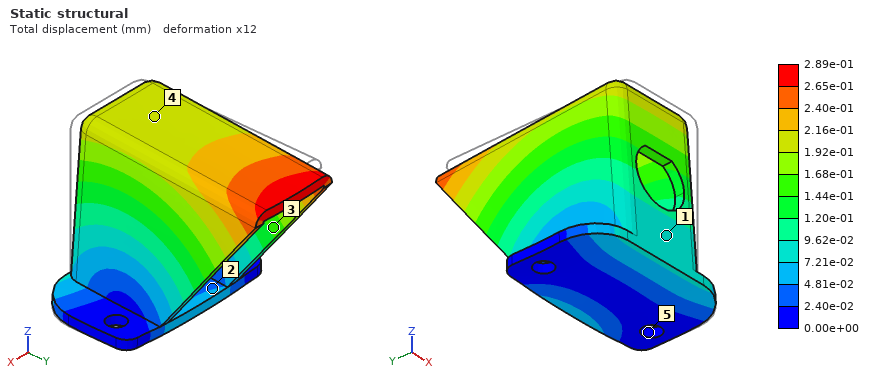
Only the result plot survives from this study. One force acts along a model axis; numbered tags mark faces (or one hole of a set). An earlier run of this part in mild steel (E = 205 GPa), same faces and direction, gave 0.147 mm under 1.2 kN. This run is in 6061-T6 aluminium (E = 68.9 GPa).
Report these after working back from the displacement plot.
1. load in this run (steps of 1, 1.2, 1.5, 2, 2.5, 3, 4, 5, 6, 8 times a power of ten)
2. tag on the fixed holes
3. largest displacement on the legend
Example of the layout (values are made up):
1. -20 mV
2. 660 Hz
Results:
1. 800 N
2. 5
3. 2.89e-01 mm
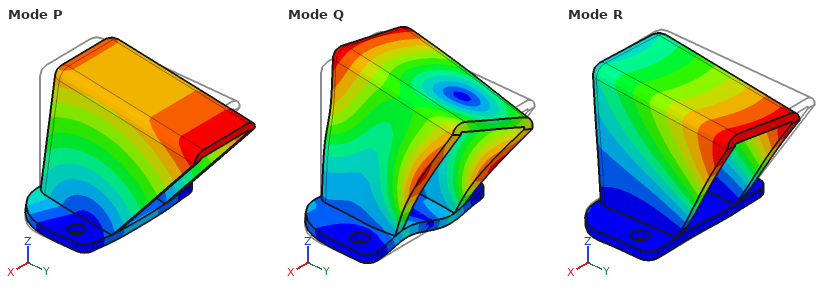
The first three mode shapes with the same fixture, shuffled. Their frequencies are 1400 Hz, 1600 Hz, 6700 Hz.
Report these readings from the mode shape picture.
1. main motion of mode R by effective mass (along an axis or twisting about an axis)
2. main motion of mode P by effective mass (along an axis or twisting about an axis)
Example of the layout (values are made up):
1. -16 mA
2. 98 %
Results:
1. along X
2. along Y
